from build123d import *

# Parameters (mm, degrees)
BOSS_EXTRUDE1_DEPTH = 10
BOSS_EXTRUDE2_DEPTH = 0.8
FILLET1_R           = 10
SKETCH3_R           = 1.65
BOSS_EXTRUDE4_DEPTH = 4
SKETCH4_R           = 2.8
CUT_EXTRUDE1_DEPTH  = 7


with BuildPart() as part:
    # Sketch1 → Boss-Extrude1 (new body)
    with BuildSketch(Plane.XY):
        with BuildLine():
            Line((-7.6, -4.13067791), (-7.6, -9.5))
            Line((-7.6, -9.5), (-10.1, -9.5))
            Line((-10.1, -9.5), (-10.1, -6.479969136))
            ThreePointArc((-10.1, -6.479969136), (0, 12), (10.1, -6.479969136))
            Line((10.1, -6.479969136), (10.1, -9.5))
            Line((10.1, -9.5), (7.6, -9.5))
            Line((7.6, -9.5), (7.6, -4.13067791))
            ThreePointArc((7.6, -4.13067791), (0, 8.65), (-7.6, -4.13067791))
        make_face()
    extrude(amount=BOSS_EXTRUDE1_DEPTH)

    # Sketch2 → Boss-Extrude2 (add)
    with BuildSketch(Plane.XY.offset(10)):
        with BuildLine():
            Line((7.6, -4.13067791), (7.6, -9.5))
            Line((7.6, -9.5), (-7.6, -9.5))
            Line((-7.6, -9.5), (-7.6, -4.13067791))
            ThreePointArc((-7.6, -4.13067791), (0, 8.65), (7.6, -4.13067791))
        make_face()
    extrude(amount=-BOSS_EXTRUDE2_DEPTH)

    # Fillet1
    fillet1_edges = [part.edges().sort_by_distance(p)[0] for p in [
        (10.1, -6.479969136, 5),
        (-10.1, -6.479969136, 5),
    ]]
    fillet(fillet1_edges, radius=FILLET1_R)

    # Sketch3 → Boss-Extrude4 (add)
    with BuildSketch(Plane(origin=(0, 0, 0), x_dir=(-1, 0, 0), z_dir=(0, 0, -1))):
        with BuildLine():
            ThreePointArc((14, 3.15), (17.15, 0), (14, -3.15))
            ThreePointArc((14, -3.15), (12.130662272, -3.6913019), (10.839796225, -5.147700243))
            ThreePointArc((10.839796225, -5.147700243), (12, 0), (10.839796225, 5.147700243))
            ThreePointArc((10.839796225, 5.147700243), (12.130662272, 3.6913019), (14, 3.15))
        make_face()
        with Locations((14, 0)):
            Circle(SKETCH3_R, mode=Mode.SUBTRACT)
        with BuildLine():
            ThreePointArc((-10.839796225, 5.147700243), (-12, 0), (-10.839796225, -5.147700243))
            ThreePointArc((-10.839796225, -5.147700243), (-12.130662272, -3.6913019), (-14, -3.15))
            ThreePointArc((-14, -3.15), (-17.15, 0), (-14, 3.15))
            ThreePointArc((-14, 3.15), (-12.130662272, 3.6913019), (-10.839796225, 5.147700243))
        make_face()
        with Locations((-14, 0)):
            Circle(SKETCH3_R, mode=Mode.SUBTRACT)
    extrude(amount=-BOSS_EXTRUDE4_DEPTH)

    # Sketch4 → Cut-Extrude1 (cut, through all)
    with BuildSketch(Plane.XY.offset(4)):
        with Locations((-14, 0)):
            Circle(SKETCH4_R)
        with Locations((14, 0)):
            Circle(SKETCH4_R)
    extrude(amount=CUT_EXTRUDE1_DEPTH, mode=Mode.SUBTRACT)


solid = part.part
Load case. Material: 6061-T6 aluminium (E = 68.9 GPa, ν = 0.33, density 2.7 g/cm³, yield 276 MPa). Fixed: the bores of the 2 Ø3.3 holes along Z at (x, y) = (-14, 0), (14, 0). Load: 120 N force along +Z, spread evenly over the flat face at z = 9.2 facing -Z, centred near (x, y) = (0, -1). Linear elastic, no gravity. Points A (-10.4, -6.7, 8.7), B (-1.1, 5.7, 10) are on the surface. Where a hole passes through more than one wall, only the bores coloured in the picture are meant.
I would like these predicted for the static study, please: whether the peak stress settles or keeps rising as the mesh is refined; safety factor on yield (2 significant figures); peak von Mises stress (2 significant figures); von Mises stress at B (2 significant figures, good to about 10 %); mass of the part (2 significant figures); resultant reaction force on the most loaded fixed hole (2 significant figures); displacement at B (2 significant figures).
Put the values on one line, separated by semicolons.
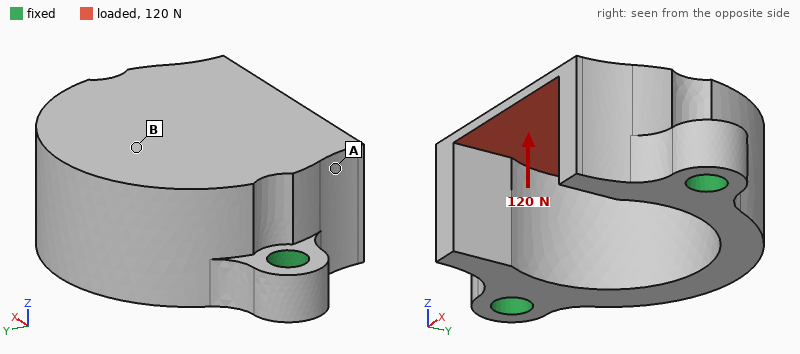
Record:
settles; 4.2; 65 MPa; 17 MPa; 5.5 g; 73 N; 6.4 µm
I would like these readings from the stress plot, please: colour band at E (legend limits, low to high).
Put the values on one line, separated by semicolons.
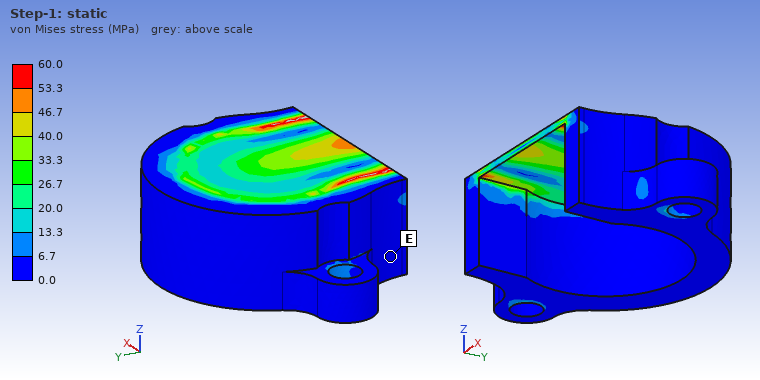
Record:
0.0 to 6.7 MPa
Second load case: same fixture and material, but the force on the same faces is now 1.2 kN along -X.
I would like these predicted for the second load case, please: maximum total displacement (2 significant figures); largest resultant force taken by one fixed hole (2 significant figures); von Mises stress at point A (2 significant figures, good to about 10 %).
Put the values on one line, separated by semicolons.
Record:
64 µm; 630 N; 23 MPa
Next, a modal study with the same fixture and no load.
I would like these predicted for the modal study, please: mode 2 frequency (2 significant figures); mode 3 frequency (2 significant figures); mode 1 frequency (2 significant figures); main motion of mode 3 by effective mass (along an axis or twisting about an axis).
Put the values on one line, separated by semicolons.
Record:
17 kHz; 19 kHz; 12 kHz; along X
